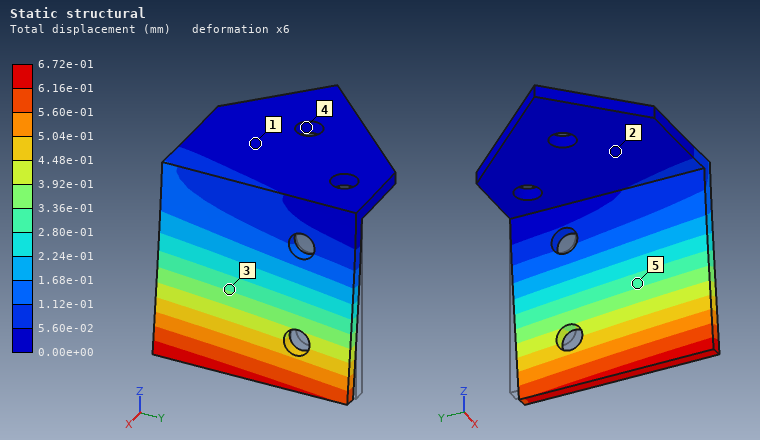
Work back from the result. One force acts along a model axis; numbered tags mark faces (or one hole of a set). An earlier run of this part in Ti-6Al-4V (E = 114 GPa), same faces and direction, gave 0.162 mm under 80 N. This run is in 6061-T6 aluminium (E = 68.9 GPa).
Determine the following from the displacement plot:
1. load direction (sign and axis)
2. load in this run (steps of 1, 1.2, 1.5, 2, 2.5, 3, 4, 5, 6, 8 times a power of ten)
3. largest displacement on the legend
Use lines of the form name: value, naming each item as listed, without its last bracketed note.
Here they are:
load direction: +X
load in this run: 200 N
largest displacement on the legend: 6.72e-01 mm
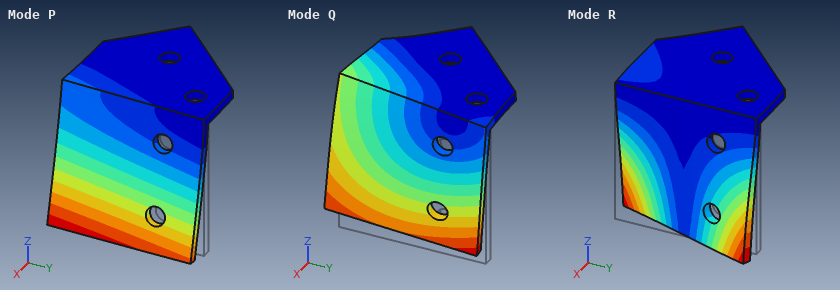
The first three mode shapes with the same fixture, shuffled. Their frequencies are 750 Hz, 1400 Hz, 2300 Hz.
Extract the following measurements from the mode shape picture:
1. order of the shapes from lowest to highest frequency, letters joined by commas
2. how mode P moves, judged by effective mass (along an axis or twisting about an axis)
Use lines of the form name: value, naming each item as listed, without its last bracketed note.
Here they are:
order of the shapes from lowest to highest frequency, letters joined by commas: P, Q, R
how mode P moves, judged by effective mass: along X
